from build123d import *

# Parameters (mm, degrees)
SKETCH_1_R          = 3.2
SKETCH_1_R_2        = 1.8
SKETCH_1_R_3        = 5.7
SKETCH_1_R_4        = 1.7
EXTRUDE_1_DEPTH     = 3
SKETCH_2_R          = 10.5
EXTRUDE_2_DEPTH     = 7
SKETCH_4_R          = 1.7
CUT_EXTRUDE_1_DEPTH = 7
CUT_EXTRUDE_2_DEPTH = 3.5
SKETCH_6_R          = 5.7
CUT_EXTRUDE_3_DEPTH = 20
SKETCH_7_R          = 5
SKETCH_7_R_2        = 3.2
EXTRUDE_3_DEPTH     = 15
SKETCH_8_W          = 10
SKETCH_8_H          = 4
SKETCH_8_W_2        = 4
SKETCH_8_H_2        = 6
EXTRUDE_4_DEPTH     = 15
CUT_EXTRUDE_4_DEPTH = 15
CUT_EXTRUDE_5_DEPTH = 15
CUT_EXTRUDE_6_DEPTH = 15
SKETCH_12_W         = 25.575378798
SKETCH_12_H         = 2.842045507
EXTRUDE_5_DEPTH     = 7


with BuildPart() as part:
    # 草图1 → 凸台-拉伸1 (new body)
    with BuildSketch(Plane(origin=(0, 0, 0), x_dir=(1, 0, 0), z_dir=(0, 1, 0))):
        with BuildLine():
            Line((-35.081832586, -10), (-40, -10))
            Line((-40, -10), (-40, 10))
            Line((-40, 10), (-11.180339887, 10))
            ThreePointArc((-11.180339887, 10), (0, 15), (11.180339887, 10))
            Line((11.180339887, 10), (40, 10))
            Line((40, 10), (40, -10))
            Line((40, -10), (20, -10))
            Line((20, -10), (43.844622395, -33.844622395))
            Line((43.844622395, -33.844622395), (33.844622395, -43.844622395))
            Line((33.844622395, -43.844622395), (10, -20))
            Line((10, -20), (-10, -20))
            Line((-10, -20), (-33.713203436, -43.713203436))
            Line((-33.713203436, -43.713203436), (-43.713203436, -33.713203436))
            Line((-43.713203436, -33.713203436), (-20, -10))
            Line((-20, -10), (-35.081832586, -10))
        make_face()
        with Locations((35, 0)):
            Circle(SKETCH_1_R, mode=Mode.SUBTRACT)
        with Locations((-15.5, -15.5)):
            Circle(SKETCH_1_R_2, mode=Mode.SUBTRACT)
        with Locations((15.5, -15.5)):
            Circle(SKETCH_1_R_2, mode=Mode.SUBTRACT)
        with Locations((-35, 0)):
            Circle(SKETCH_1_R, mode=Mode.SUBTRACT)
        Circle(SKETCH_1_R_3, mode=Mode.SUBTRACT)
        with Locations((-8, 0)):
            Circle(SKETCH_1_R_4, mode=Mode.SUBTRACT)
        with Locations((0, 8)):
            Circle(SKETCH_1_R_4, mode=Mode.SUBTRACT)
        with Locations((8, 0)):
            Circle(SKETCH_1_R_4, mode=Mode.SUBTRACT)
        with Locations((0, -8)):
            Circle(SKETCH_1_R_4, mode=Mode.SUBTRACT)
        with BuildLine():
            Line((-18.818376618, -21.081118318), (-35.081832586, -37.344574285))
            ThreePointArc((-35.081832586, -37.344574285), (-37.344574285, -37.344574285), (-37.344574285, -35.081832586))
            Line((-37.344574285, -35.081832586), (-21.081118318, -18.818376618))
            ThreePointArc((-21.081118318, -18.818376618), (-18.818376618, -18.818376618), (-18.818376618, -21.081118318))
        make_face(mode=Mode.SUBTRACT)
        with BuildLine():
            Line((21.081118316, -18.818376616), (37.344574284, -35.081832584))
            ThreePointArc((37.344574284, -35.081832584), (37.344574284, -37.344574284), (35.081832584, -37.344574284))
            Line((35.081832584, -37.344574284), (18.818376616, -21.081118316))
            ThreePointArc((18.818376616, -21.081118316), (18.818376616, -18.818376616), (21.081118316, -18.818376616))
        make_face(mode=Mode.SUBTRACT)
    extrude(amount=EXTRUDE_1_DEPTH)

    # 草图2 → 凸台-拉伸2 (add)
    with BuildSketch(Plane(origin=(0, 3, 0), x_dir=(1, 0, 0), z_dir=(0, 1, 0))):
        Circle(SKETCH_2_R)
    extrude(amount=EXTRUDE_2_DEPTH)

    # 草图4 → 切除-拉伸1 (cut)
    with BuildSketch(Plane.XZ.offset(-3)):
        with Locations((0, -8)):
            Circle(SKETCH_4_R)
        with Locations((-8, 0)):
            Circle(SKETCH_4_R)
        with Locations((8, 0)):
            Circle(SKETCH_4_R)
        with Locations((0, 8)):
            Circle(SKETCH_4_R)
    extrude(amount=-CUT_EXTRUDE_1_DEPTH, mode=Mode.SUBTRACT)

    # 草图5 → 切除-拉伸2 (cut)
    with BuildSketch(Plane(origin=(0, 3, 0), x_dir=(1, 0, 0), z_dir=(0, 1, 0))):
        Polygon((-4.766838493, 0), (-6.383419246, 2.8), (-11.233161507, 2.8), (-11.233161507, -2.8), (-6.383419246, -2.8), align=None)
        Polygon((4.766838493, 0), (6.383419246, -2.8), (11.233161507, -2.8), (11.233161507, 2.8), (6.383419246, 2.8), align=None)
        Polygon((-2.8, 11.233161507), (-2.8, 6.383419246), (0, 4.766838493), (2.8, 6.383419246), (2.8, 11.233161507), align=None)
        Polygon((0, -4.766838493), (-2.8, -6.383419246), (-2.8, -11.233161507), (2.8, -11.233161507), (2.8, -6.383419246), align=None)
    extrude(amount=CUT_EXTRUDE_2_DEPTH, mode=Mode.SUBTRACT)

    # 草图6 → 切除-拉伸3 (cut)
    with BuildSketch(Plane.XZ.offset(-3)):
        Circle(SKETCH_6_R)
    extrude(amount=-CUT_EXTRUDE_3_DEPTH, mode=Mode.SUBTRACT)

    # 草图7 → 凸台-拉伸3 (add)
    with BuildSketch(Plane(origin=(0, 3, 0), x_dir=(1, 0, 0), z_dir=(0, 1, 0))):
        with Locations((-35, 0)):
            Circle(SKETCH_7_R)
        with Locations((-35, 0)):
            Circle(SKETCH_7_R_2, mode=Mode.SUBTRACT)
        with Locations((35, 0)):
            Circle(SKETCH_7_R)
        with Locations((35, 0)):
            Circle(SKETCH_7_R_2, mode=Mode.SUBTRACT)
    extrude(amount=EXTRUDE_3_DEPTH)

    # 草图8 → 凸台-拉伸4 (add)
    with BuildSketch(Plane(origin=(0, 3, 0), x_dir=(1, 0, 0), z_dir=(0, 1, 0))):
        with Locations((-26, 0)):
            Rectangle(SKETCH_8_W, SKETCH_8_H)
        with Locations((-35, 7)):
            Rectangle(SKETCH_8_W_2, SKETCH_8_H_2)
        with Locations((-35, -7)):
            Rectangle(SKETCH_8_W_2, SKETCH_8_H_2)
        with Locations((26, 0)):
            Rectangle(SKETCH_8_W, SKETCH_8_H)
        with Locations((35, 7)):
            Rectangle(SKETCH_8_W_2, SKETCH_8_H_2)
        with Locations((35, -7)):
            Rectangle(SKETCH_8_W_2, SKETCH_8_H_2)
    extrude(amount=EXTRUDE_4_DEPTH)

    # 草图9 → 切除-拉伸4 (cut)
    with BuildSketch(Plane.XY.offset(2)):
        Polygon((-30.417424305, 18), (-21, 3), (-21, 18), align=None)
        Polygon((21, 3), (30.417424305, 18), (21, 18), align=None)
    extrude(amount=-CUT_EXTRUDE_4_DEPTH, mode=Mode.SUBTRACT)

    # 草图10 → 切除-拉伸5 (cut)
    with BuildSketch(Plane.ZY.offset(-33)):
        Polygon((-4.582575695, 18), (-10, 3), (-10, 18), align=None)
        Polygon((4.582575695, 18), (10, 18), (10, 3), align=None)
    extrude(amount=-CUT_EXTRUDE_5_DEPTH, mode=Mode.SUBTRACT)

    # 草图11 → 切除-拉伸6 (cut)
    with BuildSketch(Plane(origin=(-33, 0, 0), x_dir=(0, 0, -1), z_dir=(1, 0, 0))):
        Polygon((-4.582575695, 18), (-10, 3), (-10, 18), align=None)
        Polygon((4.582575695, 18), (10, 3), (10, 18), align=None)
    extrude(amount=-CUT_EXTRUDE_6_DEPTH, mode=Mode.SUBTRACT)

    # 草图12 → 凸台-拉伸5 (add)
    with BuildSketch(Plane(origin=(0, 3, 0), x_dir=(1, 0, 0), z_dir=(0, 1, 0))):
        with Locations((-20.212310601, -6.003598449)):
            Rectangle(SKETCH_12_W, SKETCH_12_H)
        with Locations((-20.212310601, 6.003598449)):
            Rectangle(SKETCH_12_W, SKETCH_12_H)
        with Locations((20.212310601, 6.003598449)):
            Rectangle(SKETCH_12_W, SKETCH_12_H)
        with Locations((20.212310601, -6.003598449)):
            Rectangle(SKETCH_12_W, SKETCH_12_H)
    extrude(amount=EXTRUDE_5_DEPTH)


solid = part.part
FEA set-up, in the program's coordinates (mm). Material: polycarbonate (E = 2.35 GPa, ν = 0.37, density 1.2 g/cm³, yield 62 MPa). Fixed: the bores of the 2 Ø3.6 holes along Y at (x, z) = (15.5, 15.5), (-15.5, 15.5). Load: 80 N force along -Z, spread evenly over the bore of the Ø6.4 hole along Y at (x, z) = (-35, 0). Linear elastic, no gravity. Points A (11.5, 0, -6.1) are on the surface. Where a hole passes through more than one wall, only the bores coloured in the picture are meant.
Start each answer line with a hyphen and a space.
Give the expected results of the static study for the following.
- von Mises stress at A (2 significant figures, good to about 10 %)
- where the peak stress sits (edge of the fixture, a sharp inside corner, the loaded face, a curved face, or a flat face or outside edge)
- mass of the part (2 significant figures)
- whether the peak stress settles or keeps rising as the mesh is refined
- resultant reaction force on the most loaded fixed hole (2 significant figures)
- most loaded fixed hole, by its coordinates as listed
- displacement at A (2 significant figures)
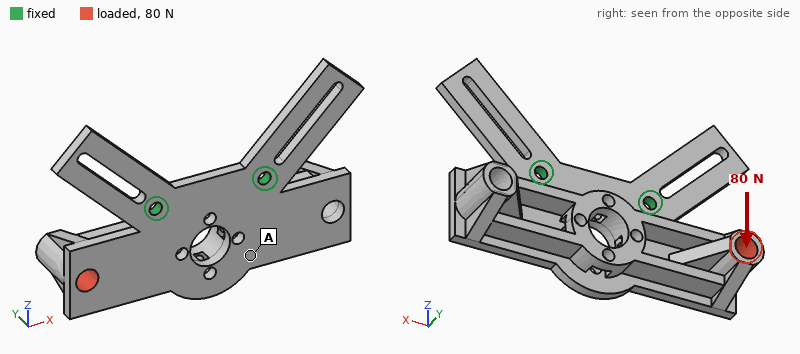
- 2.2 MPa
- edge of the fixture
- 16 g
- keeps rising
- 130 N
- (-15.5, 15.5)
- 0.38 mm
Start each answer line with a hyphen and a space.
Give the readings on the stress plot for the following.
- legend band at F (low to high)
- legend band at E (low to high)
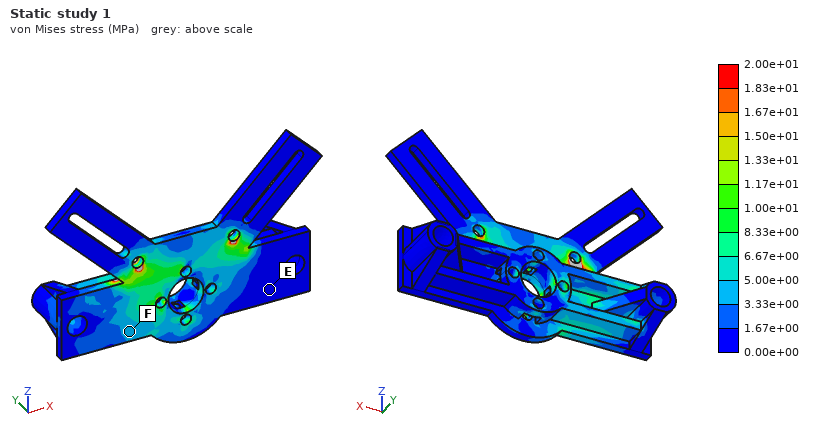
- 3.33e+00 to 5.00e+00 MPa
- 0.00e+00 to 1.67e+00 MPa
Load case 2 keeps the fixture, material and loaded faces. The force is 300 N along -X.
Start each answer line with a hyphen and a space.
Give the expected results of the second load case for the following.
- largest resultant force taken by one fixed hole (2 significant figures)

- 210 N
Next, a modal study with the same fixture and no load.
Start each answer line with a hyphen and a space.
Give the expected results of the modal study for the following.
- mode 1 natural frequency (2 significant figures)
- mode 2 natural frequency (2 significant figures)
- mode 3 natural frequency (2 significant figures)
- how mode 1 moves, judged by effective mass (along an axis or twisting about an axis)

- 480 Hz
- 630 Hz
- 650 Hz
- along Y
